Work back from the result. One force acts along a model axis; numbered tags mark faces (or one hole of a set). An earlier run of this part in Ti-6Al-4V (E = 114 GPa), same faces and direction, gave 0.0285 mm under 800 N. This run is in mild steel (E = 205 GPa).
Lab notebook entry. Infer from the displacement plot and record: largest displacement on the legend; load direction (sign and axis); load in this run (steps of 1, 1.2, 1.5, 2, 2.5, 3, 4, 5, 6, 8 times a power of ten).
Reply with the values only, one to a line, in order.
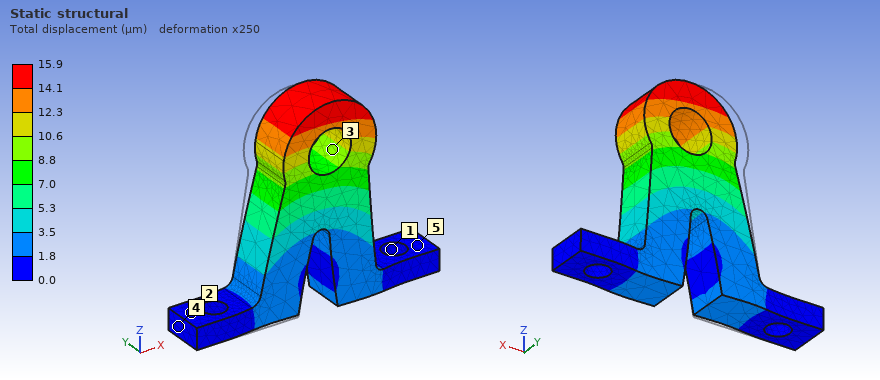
15.9 µm
+X
800 N
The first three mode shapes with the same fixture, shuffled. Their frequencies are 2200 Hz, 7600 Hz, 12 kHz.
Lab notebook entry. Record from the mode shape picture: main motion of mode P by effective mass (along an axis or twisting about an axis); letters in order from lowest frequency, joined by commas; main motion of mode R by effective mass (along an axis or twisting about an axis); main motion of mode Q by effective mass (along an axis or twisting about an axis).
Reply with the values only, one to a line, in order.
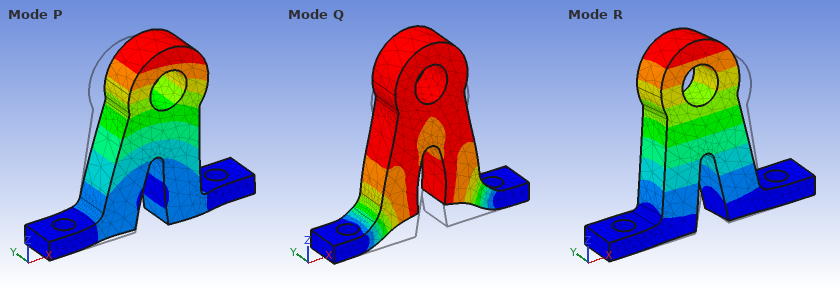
along X
R, P, Q
along Y
along Z
